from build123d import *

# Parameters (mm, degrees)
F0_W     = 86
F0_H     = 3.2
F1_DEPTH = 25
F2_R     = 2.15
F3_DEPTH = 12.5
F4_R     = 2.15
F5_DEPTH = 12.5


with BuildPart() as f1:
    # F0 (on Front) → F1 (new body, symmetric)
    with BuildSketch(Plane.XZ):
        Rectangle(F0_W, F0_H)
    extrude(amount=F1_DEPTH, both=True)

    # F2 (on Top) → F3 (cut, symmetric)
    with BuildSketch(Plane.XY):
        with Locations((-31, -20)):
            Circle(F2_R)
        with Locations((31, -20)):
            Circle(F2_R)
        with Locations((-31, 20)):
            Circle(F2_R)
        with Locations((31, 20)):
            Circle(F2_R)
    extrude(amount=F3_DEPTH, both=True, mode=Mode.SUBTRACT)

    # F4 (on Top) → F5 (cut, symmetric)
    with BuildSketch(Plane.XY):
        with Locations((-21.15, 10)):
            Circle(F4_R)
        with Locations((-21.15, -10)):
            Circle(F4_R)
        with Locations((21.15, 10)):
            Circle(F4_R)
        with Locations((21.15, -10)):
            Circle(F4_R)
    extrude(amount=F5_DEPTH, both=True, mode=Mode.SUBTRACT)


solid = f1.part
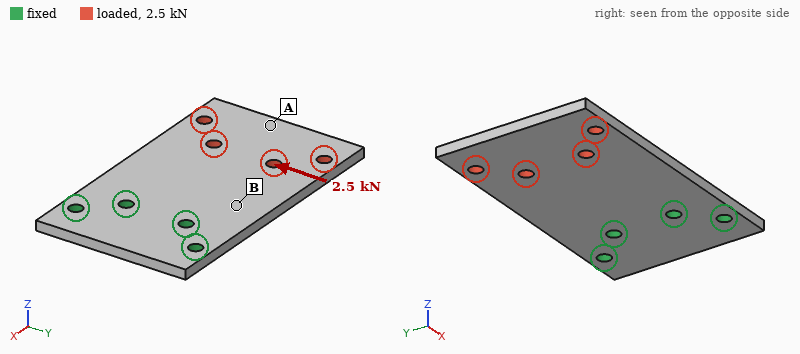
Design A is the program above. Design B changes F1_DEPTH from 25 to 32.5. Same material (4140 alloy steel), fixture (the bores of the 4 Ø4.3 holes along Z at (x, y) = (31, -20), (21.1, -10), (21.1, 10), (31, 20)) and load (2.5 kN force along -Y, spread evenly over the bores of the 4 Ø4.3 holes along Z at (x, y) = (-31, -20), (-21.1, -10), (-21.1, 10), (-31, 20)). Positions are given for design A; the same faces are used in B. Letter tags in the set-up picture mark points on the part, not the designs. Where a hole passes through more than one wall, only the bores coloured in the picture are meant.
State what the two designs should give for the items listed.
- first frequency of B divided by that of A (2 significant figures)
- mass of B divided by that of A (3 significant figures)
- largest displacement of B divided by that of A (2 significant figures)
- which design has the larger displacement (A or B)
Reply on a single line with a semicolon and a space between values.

0.97; 1.31; 0.70; A
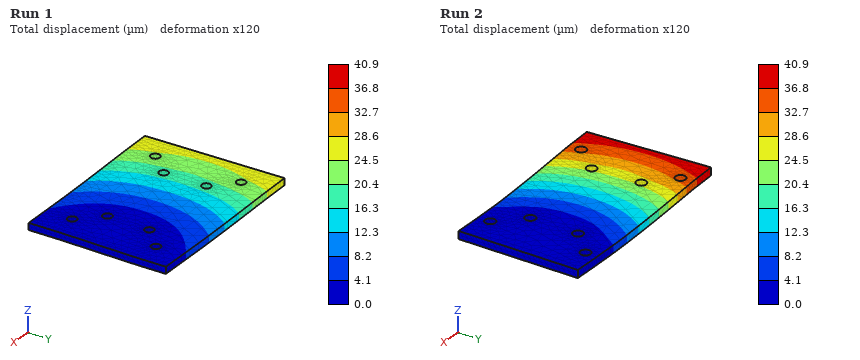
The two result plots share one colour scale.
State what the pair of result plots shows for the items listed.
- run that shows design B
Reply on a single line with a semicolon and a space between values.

Run 1
